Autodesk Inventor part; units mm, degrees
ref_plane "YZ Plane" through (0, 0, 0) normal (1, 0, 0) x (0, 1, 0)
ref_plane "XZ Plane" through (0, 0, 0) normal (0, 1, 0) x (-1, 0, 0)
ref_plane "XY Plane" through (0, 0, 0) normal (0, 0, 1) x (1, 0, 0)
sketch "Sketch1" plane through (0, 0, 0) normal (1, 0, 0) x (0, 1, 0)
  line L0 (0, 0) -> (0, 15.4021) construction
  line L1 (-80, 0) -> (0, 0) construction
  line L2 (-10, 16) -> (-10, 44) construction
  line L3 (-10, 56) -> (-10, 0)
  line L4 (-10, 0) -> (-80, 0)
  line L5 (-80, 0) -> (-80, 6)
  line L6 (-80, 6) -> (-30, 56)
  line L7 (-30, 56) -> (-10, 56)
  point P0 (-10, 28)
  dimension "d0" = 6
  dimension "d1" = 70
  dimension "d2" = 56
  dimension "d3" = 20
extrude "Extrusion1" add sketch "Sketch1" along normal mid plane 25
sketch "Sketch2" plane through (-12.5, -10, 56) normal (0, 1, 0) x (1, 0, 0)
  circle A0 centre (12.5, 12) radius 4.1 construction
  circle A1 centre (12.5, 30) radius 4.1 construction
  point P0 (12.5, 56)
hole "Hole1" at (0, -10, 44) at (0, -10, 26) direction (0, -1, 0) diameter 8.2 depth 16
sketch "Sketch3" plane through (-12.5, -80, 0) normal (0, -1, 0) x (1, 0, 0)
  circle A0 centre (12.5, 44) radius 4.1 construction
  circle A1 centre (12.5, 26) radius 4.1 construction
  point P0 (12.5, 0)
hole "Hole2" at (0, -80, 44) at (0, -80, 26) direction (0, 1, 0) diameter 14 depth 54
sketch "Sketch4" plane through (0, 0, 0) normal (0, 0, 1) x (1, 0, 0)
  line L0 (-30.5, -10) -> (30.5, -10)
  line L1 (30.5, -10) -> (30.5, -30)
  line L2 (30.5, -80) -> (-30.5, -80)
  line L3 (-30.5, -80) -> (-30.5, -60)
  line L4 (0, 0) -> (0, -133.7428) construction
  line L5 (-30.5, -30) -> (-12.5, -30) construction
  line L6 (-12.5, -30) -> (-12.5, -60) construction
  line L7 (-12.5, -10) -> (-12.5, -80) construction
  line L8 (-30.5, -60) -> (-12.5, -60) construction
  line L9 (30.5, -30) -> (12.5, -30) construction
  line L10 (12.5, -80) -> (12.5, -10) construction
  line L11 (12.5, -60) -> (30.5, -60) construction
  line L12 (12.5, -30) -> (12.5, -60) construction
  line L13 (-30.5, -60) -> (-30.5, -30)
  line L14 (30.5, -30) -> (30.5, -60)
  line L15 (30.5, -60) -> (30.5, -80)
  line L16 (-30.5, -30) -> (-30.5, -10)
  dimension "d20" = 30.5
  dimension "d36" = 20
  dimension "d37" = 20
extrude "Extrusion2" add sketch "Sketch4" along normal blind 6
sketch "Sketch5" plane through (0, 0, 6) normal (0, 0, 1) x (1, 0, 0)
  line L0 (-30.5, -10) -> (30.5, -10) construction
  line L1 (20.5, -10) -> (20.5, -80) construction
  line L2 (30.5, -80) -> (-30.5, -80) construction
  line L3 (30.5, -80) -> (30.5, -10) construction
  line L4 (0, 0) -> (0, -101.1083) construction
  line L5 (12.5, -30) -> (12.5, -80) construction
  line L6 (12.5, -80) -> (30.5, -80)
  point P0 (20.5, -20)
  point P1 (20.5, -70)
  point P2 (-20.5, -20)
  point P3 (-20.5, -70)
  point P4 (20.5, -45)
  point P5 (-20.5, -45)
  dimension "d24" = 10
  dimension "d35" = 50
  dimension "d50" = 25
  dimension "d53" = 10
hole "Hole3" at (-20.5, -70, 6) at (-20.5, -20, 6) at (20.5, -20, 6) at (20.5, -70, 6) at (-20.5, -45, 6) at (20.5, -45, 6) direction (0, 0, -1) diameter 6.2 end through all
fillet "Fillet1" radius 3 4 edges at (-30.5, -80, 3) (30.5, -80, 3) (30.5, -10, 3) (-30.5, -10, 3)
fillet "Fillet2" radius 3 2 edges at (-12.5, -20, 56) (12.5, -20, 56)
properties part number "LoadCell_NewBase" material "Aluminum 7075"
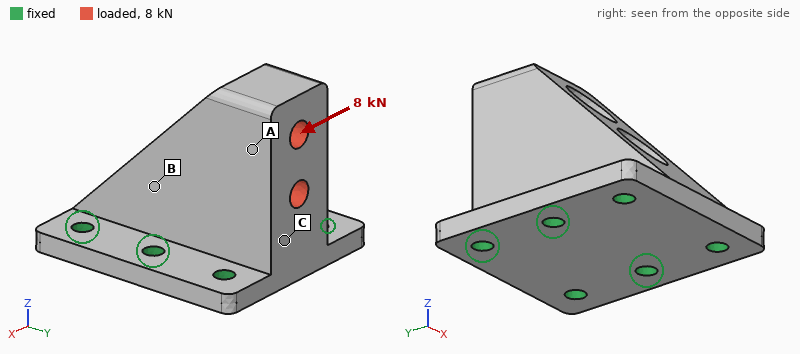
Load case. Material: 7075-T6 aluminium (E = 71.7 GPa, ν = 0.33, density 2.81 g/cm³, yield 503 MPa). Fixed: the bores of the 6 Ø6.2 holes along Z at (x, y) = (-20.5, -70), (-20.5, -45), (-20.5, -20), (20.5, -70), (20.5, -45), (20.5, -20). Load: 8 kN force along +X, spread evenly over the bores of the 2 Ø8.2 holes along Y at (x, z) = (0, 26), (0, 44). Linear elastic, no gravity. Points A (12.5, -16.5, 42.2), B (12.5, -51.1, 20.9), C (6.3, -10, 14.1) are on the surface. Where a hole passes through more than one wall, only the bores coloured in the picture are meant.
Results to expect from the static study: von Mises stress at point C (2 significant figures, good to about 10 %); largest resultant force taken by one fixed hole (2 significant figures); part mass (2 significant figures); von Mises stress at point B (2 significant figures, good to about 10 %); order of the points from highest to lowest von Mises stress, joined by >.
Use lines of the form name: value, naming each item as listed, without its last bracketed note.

von Mises stress at point C: 32 MPa
largest resultant force taken by one fixed hole: 4.6 kN
part mass: 200 g
von Mises stress at point B: 44 MPa
order of the points from highest to lowest von Mises stress, joined by >: B > C > A
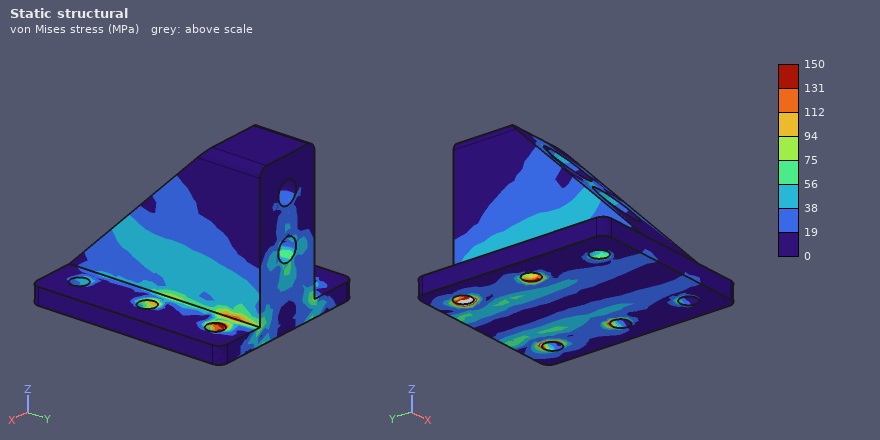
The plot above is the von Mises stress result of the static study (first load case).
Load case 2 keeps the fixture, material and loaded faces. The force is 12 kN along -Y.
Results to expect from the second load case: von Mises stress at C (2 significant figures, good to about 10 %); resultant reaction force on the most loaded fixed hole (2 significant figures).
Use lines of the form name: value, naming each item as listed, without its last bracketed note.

von Mises stress at C: 24 MPa
resultant reaction force on the most loaded fixed hole: 4.7 kN
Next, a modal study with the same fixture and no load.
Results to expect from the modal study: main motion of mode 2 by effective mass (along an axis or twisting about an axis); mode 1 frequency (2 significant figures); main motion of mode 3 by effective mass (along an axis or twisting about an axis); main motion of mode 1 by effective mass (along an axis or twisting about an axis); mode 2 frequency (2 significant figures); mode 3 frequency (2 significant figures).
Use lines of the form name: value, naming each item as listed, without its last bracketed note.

main motion of mode 2 by effective mass: along Y
mode 1 frequency: 5500 Hz
main motion of mode 3 by effective mass: along Z
main motion of mode 1 by effective mass: along X
mode 2 frequency: 6600 Hz
mode 3 frequency: 12 kHz
